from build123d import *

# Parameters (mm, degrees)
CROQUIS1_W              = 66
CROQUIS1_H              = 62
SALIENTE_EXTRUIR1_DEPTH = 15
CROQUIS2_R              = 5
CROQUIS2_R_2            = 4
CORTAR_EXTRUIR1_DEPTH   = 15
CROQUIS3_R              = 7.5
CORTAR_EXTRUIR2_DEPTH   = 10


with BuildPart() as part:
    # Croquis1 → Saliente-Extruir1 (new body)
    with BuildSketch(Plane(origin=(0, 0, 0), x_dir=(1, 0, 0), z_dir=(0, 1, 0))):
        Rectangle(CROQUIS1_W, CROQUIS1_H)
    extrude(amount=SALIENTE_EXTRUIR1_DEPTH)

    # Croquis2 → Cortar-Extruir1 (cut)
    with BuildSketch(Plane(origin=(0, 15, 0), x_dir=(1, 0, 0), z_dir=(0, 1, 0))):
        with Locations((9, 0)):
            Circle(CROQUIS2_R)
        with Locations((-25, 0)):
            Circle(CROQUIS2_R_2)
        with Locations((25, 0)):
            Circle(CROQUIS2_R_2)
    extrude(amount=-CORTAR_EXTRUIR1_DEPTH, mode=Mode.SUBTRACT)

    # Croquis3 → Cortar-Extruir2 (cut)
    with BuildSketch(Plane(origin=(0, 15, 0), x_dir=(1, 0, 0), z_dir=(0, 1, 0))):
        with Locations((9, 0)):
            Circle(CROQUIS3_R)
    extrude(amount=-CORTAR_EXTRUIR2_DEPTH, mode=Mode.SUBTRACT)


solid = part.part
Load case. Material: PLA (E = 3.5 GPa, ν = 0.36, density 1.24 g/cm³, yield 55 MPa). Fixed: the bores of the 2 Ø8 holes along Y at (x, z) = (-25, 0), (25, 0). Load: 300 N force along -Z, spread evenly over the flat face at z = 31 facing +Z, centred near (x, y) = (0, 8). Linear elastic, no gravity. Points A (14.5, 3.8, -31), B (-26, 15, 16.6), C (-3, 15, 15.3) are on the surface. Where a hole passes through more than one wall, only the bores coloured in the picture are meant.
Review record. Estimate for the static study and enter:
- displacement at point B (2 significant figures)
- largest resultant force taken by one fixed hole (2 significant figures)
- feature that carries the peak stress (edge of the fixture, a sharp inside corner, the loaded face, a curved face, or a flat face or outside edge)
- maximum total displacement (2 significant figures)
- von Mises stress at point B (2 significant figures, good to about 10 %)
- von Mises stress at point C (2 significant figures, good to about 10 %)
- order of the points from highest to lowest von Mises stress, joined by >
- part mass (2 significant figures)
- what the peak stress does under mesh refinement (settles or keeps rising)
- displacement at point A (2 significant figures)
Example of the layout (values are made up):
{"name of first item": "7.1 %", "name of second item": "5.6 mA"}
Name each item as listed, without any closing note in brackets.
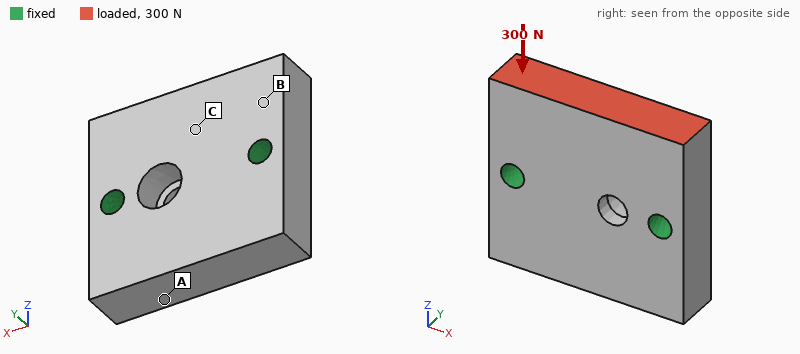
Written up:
{"displacement at point B": "1.8 µm", "largest resultant force taken by one fixed hole": "150 N", "feature that carries the peak stress": "edge of the fixture", "maximum total displacement": "4.0 µm", "von Mises stress at point B": "0.37 MPa", "von Mises stress at point C": "0.23 MPa", "order of the points from highest to lowest von Mises stress, joined by >": "B > C > A", "part mass": "72 g", "what the peak stress does under mesh refinement": "keeps rising", "displacement at point A": "0.85 µm"}
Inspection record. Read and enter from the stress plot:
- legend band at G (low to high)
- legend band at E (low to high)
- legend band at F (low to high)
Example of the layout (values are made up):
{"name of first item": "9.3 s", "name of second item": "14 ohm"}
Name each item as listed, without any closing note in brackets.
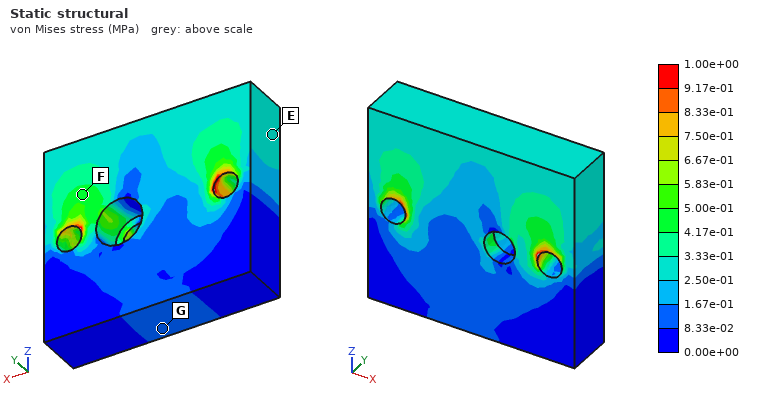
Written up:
{"legend band at G": "8.33e-02 to 1.67e-01 MPa", "legend band at E": "2.50e-01 to 3.33e-01 MPa", "legend band at F": "4.17e-01 to 5.00e-01 MPa"}
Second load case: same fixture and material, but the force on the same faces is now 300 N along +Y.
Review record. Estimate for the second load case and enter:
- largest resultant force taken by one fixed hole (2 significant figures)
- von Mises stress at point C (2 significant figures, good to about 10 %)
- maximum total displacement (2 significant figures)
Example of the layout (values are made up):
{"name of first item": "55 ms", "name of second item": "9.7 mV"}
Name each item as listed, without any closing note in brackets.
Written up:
{"largest resultant force taken by one fixed hole": "160 N", "von Mises stress at point C": "1.6 MPa", "maximum total displacement": "76 µm"}
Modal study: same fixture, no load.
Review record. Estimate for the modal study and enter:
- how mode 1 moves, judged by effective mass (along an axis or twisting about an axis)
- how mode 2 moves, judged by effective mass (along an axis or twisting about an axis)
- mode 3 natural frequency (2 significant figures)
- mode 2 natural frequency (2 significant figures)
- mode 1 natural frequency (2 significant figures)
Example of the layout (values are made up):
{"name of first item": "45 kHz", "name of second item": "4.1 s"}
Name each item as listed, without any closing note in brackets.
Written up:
{"how mode 1 moves, judged by effective mass": "twisting about X", "how mode 2 moves, judged by effective mass": "along Y", "mode 3 natural frequency": "5000 Hz", "mode 2 natural frequency": "3500 Hz", "mode 1 natural frequency": "2900 Hz"}
